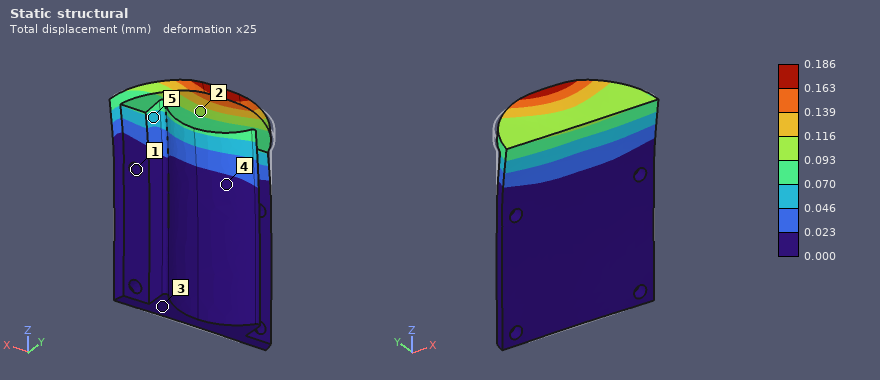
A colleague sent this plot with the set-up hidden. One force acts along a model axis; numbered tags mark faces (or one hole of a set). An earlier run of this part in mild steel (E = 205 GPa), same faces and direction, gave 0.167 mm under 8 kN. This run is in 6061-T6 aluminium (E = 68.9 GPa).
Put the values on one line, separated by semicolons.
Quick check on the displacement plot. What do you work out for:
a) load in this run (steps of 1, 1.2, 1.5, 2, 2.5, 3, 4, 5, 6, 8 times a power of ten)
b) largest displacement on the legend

3 kN; 0.186 mm
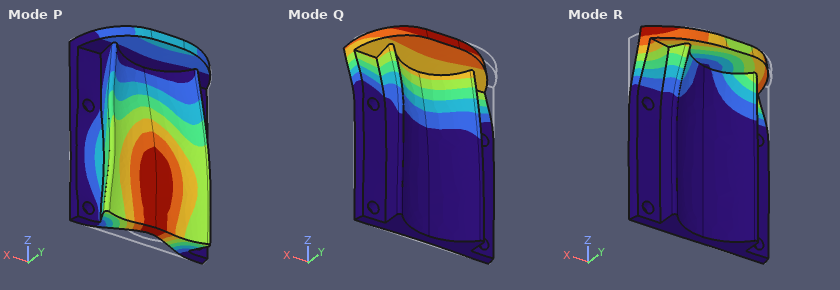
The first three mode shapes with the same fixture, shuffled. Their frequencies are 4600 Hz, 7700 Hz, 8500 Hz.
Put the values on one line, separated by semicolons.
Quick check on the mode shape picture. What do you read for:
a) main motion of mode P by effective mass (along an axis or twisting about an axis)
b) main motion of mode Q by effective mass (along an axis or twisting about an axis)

along Y; along Y
